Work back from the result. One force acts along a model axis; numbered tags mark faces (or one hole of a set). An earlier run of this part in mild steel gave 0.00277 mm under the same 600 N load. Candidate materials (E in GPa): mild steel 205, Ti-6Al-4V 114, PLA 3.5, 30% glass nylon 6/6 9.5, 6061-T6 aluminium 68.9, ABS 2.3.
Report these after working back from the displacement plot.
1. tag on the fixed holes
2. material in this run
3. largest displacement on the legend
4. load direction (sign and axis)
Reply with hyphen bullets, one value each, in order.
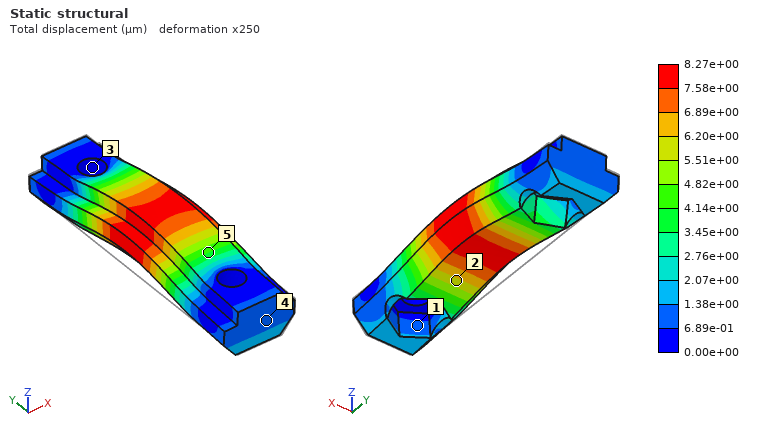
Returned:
- 3
- 6061-T6 aluminium
- 8.27e+00 µm
- +Z
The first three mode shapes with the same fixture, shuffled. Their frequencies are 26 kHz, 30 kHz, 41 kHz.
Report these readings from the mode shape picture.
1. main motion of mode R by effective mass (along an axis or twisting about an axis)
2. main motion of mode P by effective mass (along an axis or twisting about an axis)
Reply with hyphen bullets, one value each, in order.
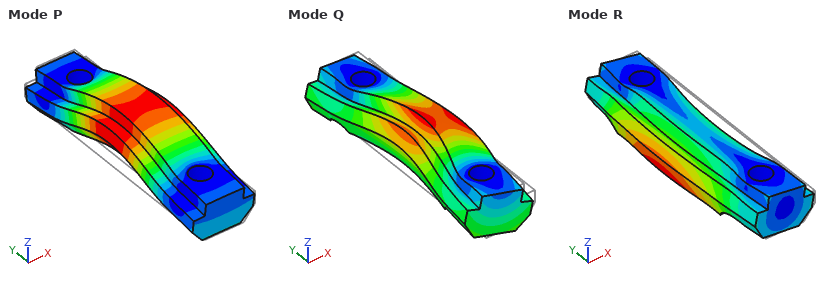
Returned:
- along X
- along Z
